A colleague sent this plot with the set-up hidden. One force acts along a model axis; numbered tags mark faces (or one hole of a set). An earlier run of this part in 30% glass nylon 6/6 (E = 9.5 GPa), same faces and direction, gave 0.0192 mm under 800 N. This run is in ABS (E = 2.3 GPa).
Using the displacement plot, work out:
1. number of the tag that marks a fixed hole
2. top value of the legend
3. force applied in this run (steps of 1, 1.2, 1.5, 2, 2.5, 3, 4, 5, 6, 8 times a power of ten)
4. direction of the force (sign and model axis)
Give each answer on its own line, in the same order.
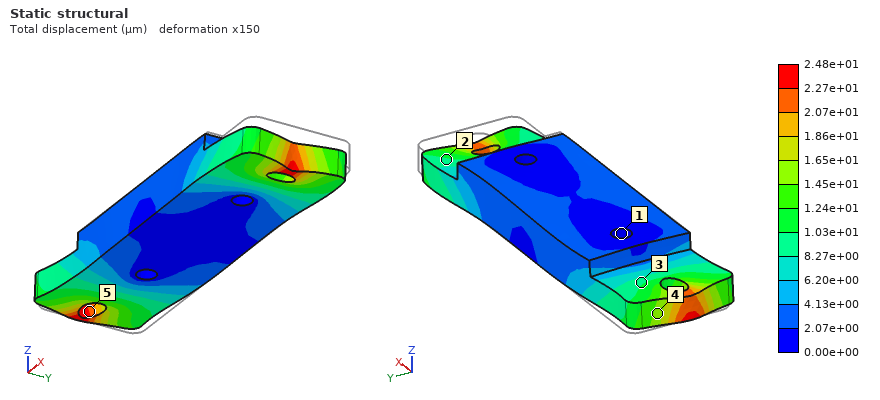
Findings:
1
2.48e+01 µm
250 N
-X
